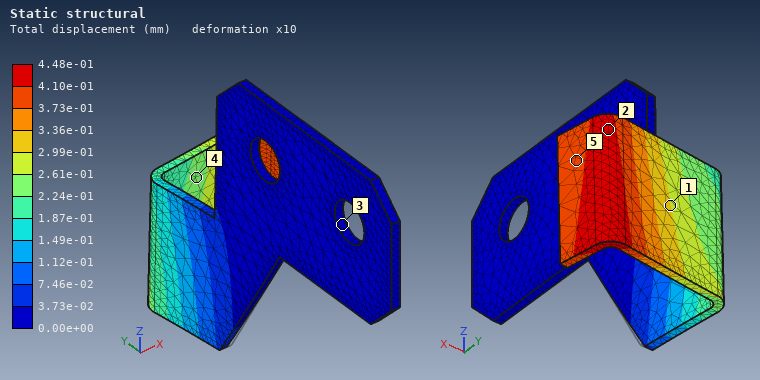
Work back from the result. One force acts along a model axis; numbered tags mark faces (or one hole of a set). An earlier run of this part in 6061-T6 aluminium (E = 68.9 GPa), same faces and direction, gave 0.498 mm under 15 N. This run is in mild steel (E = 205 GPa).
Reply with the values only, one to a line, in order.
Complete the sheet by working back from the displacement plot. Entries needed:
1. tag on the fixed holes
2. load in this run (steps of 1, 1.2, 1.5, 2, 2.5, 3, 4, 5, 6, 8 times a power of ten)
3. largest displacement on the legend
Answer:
3
40 N
4.48e-01 mm
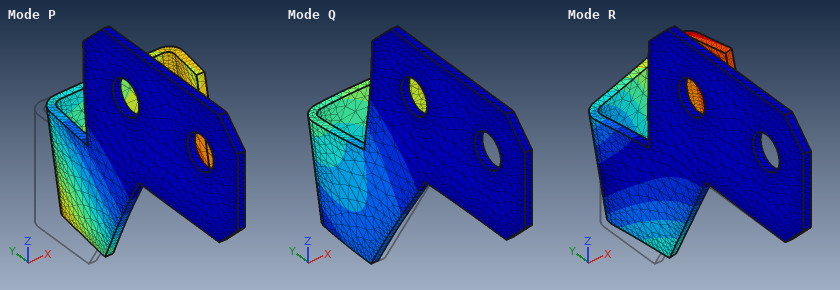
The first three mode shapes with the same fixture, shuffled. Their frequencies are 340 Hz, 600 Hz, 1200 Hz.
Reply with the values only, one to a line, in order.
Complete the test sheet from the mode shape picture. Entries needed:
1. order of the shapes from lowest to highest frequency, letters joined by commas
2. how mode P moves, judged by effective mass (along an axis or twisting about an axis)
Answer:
P, R, Q
along X
